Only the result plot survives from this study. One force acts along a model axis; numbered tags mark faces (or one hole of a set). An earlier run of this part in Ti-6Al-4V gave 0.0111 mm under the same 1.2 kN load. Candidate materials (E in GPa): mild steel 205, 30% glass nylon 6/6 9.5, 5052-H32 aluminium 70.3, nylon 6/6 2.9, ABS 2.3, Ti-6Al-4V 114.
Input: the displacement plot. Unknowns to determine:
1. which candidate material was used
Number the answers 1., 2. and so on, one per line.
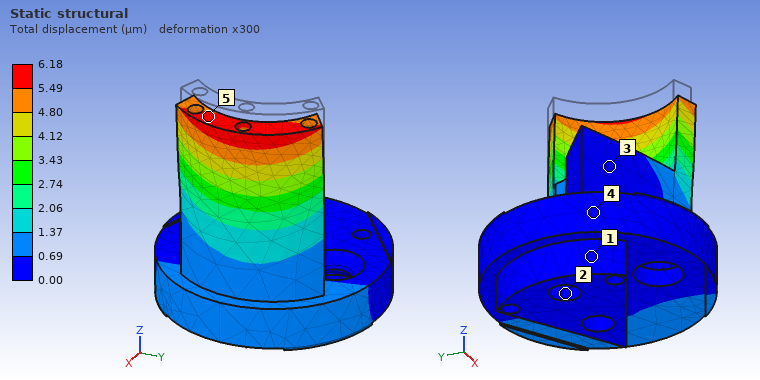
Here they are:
1. mild steel
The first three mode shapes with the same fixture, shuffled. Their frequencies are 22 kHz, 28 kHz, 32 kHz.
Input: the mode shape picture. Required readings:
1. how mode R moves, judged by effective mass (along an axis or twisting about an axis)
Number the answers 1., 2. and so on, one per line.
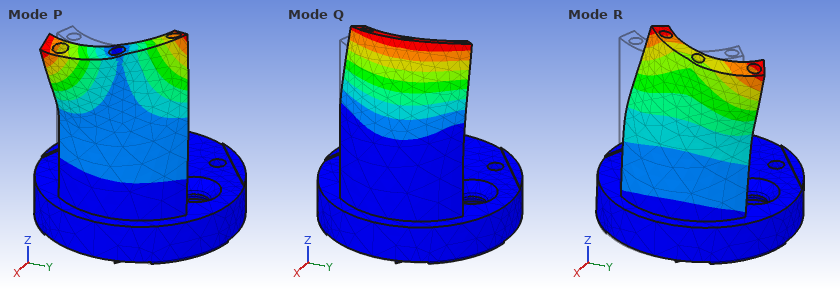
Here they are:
1. along Y
